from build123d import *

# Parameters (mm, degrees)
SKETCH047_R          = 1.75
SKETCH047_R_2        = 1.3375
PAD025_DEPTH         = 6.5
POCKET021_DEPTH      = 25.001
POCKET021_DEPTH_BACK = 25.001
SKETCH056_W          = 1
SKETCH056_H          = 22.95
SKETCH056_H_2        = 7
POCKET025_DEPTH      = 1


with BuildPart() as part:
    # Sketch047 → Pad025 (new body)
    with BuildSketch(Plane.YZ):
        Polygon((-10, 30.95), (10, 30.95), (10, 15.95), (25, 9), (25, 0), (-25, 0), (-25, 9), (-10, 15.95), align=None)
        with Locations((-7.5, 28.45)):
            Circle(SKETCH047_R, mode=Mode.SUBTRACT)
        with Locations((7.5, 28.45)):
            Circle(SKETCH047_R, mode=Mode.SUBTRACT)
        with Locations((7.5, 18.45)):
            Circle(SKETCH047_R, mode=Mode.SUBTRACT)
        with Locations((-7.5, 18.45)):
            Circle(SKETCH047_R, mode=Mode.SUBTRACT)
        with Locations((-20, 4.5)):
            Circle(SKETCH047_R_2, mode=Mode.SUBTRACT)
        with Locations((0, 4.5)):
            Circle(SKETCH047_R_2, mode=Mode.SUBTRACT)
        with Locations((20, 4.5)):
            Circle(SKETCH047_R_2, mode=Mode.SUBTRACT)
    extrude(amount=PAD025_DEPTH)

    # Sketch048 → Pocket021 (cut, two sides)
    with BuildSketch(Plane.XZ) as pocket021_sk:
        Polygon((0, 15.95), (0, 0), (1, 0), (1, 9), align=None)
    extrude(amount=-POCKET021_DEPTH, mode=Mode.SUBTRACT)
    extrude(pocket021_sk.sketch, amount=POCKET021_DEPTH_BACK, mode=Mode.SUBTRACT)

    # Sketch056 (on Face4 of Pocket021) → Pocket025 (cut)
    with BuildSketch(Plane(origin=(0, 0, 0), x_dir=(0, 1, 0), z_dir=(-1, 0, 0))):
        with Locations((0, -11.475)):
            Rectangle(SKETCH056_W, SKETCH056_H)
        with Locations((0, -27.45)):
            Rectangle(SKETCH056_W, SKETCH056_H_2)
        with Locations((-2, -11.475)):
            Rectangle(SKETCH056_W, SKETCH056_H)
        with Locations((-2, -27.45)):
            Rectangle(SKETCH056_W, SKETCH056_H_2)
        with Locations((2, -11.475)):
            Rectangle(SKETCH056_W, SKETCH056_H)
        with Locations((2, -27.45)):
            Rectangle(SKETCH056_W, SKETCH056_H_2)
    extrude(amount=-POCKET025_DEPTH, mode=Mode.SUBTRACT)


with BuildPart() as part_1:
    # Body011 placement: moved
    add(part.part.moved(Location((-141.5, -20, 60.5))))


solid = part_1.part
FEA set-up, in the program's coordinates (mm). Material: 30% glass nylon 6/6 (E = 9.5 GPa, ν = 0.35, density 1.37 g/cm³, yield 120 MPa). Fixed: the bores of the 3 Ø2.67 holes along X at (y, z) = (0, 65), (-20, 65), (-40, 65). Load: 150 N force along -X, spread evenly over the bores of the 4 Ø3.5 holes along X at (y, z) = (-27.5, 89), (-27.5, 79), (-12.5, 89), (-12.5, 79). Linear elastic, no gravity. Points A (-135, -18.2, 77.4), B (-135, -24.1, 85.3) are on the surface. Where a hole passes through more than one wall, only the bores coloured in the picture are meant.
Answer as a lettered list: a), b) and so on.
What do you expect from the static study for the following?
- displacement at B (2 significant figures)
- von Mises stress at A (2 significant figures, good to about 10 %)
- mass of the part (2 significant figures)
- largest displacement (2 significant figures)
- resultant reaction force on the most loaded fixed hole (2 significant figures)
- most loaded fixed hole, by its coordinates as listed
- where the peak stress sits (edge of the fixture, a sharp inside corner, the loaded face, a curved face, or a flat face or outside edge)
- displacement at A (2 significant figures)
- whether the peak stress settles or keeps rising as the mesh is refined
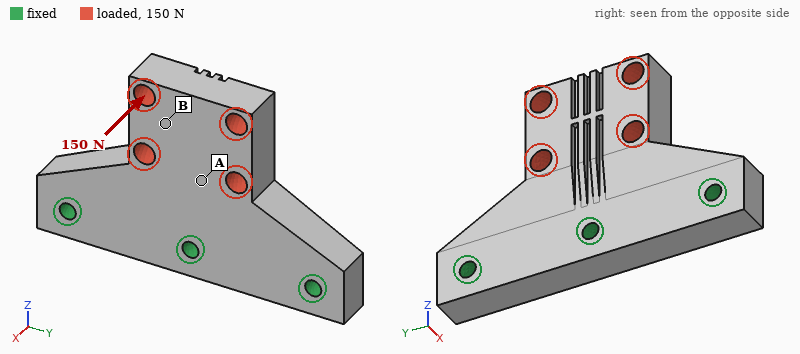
a) 0.13 mm
b) 8.2 MPa
c) 7.5 g
d) 0.19 mm
e) 120 N
f) (-20, 65)
g) edge of the fixture
h) 0.066 mm
i) keeps rising
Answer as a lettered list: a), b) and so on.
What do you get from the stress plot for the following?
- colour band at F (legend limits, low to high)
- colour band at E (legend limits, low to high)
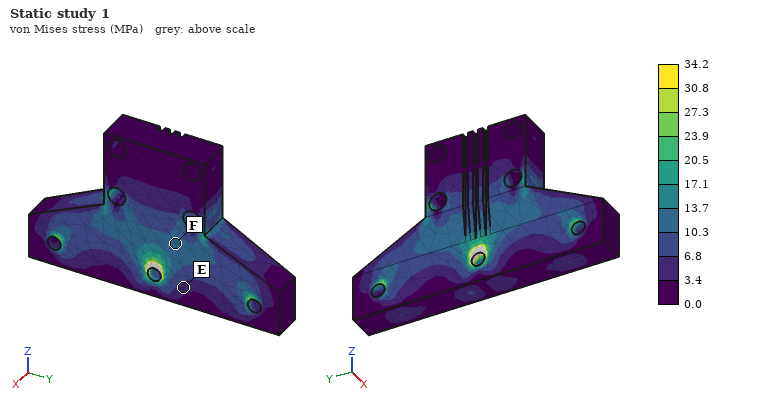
a) 10.3 to 13.7 MPa
b) 3.4 to 6.8 MPa
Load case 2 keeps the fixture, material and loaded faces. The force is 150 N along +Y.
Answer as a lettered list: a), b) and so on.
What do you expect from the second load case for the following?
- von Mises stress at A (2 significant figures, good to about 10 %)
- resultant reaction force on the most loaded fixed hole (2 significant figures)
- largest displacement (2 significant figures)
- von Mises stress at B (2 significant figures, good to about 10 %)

a) 2.0 MPa
b) 92 N
c) 18 µm
d) 0.89 MPa
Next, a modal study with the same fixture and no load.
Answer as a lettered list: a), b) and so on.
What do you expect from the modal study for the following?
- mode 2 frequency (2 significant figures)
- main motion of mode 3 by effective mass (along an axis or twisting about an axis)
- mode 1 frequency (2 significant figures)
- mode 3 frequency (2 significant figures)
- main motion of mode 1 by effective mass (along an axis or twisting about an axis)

a) 9800 Hz
b) along Y
c) 3500 Hz
d) 11 kHz
e) along X
